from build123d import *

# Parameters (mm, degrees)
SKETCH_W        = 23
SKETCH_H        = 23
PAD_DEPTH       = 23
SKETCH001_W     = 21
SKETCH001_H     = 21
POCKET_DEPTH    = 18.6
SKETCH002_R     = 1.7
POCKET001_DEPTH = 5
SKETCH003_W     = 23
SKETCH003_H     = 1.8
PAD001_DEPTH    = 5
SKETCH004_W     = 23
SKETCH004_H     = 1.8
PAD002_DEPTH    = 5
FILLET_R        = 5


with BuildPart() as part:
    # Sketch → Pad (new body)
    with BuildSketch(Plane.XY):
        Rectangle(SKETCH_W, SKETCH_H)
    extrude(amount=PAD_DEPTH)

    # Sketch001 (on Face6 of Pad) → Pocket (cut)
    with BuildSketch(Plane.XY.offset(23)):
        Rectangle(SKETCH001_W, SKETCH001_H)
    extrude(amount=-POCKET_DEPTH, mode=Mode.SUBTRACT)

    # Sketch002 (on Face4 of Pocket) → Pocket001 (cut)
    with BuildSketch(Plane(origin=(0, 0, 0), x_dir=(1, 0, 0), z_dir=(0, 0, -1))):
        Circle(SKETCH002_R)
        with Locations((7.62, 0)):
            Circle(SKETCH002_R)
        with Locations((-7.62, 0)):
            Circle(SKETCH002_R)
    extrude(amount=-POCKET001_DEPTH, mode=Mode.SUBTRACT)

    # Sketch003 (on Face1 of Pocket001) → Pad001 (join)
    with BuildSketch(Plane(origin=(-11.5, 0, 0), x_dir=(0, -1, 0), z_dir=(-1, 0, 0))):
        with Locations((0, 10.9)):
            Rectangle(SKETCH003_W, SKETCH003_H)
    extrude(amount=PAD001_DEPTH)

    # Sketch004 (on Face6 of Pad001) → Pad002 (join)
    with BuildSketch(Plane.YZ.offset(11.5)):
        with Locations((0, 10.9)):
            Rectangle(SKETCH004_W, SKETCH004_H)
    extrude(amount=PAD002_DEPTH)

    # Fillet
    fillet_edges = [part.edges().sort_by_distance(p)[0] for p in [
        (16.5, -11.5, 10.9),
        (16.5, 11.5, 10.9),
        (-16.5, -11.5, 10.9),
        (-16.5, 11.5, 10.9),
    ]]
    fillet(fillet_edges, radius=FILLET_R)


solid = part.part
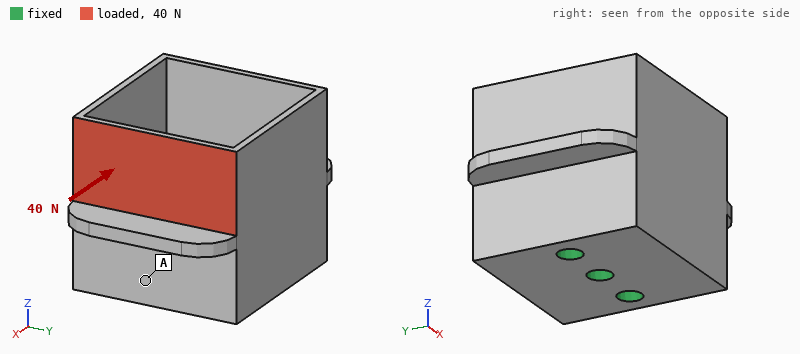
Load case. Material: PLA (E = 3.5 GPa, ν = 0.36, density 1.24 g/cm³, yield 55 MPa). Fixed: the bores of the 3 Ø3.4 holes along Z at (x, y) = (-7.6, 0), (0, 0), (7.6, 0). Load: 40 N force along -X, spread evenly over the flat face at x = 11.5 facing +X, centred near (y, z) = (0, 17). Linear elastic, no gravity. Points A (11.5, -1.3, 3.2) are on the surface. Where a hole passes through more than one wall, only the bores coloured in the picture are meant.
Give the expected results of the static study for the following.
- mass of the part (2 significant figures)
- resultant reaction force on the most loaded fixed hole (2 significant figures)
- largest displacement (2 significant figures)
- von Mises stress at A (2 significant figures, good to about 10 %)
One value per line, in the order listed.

5.2 g
33 N
0.45 mm
1.9 MPa
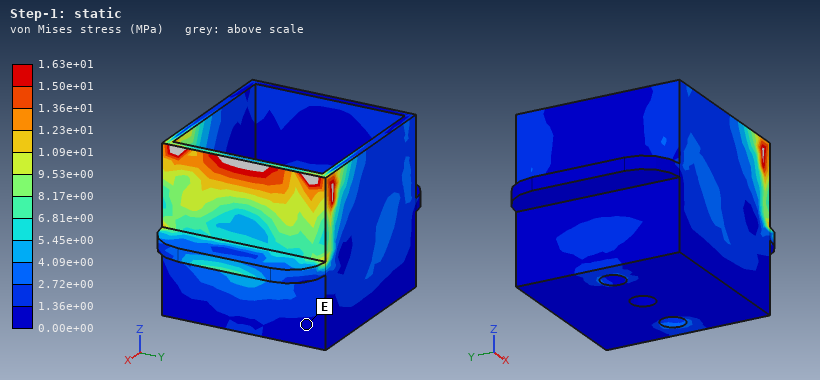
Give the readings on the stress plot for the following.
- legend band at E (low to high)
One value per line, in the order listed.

0.00e+00 to 1.36e+00 MPa
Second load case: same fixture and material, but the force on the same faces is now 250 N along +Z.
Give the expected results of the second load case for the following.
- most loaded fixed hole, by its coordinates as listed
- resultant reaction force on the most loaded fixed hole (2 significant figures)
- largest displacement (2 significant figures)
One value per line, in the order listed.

(7.6, 0)
260 N
0.32 mm
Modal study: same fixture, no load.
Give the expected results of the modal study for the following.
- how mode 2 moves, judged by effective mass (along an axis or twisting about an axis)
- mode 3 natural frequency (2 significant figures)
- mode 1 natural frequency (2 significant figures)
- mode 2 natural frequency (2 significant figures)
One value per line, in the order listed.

along Y
3300 Hz
2700 Hz
2900 Hz
